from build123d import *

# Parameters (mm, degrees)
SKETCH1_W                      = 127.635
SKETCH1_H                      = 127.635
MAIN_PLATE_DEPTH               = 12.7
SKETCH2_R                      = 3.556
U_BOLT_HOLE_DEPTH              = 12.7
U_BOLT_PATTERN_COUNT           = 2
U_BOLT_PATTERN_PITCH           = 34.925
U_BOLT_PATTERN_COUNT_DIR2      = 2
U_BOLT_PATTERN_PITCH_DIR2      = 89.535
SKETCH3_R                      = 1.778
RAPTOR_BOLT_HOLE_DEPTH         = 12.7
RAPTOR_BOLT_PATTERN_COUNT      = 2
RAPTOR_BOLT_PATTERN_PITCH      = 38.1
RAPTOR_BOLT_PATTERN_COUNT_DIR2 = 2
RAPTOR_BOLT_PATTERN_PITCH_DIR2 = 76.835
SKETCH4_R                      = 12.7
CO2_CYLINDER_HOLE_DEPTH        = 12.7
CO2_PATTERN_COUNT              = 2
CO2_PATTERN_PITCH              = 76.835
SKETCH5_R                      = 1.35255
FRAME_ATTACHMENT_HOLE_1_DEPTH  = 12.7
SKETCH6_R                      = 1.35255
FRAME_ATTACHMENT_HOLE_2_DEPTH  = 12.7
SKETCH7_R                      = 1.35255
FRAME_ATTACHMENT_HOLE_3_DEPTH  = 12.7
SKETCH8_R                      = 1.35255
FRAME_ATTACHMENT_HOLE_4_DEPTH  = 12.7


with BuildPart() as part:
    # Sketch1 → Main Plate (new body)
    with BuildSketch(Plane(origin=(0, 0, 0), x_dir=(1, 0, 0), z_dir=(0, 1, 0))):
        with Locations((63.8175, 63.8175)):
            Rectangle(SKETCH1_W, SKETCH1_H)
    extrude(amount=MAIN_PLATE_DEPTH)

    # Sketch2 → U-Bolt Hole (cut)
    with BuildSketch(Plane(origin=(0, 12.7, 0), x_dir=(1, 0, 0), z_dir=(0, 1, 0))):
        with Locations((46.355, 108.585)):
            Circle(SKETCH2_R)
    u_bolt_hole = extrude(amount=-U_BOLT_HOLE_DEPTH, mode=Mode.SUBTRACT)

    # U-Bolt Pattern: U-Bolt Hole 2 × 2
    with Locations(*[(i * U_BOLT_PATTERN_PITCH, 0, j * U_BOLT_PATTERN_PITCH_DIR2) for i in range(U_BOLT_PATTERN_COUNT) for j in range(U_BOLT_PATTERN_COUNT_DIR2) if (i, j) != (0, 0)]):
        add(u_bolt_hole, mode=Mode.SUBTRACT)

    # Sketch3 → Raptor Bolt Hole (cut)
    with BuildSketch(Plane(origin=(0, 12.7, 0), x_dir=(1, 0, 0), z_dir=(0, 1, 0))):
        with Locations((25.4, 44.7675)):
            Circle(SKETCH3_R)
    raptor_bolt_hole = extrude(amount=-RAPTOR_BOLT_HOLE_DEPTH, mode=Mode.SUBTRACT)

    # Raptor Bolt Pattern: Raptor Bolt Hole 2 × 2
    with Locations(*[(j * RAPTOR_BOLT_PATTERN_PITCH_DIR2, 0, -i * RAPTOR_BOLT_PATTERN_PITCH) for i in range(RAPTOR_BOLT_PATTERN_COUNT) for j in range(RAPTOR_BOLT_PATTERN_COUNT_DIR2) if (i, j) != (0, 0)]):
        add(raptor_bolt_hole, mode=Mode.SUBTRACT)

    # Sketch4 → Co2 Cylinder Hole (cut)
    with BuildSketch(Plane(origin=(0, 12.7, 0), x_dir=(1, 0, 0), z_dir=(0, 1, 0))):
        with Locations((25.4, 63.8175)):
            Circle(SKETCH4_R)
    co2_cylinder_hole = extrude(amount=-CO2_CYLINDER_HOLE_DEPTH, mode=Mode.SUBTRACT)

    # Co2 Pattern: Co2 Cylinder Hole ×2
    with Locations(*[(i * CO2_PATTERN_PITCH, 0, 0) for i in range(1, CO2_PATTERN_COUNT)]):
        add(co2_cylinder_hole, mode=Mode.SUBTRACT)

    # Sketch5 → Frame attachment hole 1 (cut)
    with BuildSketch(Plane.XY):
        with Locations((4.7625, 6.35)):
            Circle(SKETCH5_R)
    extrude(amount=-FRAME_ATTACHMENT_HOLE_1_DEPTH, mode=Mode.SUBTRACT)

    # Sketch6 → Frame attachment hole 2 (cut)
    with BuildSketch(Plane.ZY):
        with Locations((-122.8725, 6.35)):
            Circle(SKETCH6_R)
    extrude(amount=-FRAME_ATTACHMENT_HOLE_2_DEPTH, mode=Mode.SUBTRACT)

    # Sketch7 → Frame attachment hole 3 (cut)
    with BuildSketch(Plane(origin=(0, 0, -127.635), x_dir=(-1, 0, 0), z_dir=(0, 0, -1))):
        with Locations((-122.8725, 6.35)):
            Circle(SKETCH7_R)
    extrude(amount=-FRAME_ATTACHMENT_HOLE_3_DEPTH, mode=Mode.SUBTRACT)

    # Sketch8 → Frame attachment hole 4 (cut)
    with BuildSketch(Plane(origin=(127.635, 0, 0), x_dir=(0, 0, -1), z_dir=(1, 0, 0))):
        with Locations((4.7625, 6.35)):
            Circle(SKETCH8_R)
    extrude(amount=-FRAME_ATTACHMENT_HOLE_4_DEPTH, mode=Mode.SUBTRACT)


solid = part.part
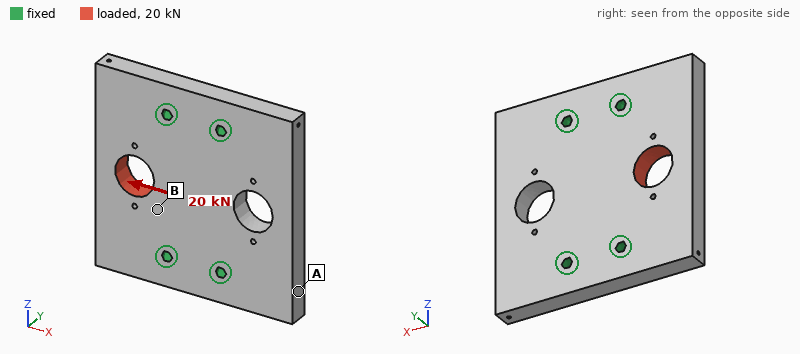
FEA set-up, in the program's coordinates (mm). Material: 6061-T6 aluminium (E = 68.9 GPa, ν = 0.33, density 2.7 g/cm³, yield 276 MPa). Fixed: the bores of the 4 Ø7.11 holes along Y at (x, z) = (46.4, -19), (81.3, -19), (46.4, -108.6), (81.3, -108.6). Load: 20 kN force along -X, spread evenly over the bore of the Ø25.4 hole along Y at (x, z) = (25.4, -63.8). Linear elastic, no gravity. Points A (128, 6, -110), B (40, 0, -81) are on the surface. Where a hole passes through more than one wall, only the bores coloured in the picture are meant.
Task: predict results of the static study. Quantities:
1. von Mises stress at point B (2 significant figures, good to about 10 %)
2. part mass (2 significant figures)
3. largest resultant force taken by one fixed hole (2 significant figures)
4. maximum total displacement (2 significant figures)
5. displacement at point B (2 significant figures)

20 MPa
520 g
6.1 kN
31 µm
13 µm
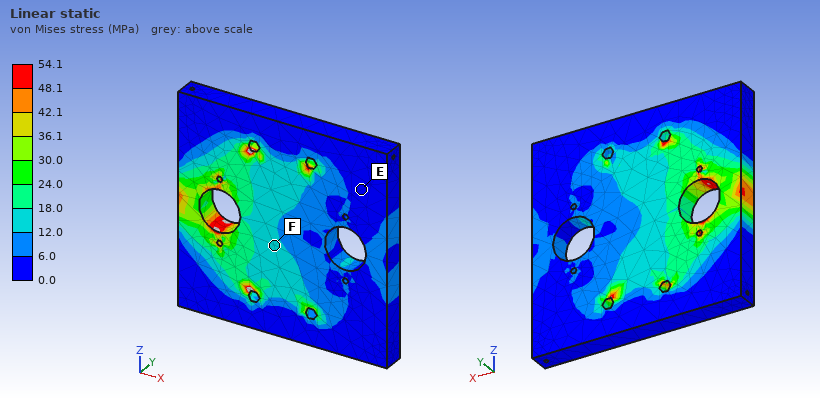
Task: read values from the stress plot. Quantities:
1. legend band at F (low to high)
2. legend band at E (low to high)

12.0 to 18.0 MPa
0.0 to 6.0 MPa
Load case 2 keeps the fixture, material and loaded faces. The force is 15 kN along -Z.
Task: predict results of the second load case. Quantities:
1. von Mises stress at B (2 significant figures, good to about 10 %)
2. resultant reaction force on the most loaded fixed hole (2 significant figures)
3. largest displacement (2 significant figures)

17 MPa
7.2 kN
23 µm
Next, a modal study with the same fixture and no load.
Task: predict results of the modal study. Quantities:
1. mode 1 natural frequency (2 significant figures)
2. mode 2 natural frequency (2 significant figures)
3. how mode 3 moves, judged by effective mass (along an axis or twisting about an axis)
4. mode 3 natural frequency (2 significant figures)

3600 Hz
3700 Hz
twisting about X
5300 Hz
